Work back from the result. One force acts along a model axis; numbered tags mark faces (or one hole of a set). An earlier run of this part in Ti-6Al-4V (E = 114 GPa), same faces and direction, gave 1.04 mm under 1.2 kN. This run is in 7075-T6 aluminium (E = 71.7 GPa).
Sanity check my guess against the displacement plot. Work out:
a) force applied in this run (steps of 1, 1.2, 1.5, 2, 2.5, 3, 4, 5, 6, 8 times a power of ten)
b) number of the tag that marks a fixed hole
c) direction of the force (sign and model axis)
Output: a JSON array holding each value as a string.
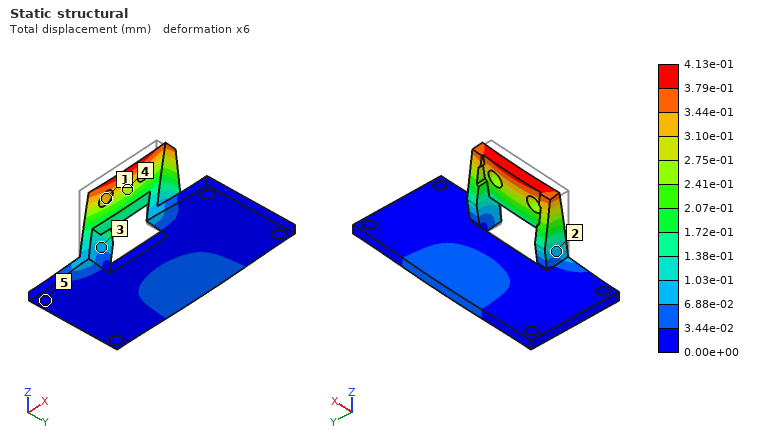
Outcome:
["300 N", "5", "+Y"]
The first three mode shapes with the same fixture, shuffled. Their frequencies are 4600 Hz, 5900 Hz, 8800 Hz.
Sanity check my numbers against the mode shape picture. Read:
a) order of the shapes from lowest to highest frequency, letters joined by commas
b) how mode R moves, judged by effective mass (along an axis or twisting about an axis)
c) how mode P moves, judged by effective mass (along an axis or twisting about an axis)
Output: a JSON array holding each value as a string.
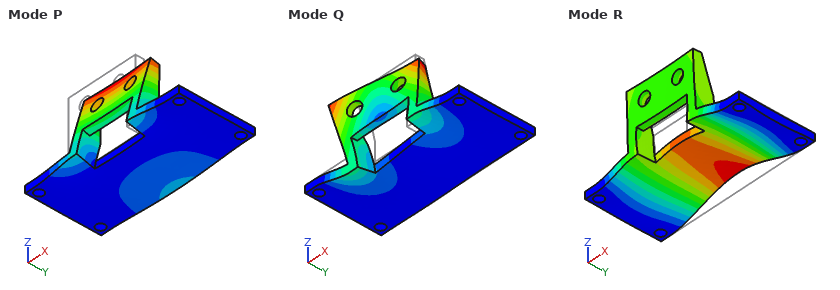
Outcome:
["P, R, Q", "along Z", "along Y"]
